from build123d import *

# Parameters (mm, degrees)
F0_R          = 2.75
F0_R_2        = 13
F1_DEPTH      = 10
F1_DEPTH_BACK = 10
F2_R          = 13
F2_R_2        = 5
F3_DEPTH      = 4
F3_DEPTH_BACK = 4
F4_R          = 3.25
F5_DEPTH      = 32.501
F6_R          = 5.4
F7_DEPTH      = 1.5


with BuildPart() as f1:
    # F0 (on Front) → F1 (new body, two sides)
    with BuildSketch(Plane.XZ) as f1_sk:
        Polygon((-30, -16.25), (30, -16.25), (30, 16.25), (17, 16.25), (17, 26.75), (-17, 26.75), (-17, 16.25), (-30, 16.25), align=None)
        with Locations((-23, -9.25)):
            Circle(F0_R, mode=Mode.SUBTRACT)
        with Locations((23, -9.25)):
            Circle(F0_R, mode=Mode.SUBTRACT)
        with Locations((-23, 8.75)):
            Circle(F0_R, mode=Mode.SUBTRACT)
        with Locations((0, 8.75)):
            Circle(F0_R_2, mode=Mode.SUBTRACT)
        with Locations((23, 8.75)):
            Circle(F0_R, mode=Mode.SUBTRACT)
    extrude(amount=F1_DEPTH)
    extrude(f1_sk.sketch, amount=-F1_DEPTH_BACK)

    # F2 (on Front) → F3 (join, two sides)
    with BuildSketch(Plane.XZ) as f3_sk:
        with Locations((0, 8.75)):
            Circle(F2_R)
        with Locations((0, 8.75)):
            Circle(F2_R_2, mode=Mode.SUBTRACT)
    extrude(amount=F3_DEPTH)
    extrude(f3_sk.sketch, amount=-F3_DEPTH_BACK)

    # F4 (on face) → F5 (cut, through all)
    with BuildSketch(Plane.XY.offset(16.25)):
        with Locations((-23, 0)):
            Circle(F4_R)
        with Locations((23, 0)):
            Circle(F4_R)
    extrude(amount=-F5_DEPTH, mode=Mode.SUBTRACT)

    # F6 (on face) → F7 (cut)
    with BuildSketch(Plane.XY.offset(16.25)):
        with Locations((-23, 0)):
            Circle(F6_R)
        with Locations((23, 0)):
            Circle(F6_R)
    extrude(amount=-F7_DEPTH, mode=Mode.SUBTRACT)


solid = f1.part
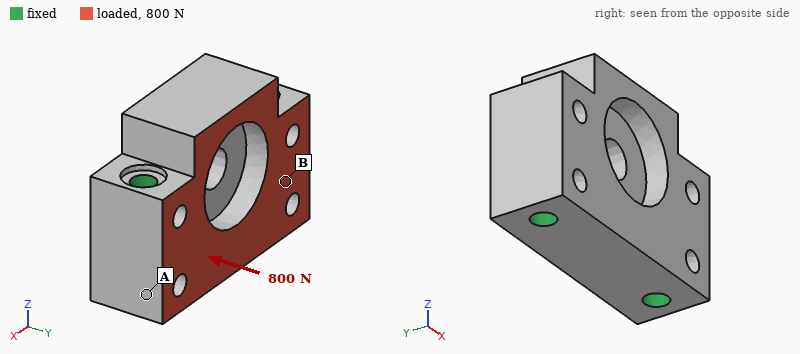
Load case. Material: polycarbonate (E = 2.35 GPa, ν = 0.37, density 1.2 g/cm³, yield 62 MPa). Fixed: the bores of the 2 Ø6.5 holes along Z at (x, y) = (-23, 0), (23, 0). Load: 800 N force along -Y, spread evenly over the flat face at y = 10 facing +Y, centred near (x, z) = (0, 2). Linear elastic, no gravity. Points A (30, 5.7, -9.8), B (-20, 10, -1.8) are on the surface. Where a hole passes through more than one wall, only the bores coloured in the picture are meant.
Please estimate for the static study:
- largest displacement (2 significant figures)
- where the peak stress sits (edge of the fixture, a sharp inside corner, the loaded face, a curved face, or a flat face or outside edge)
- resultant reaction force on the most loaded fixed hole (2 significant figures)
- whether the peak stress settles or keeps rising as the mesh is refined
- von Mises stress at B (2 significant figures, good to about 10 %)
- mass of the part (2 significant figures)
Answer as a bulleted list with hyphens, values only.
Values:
- 39 µm
- edge of the fixture
- 400 N
- keeps rising
- 0.95 MPa
- 43 g
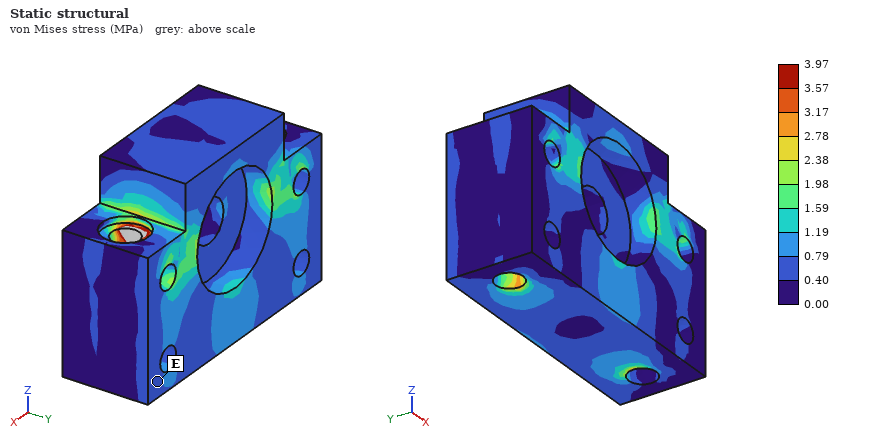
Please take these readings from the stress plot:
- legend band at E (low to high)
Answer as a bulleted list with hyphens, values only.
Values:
- 0.40 to 0.79 MPa
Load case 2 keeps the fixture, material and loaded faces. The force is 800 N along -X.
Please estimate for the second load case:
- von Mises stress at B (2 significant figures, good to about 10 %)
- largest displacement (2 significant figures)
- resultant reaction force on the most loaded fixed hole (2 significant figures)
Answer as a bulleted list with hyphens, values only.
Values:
- 0.88 MPa
- 23 µm
- 420 N
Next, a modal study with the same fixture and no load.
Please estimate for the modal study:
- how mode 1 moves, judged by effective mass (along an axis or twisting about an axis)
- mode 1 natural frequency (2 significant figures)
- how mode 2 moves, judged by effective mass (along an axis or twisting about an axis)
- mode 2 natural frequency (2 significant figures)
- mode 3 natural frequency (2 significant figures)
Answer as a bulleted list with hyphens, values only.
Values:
- along Y
- 4200 Hz
- along Y
- 6700 Hz
- 7400 Hz
